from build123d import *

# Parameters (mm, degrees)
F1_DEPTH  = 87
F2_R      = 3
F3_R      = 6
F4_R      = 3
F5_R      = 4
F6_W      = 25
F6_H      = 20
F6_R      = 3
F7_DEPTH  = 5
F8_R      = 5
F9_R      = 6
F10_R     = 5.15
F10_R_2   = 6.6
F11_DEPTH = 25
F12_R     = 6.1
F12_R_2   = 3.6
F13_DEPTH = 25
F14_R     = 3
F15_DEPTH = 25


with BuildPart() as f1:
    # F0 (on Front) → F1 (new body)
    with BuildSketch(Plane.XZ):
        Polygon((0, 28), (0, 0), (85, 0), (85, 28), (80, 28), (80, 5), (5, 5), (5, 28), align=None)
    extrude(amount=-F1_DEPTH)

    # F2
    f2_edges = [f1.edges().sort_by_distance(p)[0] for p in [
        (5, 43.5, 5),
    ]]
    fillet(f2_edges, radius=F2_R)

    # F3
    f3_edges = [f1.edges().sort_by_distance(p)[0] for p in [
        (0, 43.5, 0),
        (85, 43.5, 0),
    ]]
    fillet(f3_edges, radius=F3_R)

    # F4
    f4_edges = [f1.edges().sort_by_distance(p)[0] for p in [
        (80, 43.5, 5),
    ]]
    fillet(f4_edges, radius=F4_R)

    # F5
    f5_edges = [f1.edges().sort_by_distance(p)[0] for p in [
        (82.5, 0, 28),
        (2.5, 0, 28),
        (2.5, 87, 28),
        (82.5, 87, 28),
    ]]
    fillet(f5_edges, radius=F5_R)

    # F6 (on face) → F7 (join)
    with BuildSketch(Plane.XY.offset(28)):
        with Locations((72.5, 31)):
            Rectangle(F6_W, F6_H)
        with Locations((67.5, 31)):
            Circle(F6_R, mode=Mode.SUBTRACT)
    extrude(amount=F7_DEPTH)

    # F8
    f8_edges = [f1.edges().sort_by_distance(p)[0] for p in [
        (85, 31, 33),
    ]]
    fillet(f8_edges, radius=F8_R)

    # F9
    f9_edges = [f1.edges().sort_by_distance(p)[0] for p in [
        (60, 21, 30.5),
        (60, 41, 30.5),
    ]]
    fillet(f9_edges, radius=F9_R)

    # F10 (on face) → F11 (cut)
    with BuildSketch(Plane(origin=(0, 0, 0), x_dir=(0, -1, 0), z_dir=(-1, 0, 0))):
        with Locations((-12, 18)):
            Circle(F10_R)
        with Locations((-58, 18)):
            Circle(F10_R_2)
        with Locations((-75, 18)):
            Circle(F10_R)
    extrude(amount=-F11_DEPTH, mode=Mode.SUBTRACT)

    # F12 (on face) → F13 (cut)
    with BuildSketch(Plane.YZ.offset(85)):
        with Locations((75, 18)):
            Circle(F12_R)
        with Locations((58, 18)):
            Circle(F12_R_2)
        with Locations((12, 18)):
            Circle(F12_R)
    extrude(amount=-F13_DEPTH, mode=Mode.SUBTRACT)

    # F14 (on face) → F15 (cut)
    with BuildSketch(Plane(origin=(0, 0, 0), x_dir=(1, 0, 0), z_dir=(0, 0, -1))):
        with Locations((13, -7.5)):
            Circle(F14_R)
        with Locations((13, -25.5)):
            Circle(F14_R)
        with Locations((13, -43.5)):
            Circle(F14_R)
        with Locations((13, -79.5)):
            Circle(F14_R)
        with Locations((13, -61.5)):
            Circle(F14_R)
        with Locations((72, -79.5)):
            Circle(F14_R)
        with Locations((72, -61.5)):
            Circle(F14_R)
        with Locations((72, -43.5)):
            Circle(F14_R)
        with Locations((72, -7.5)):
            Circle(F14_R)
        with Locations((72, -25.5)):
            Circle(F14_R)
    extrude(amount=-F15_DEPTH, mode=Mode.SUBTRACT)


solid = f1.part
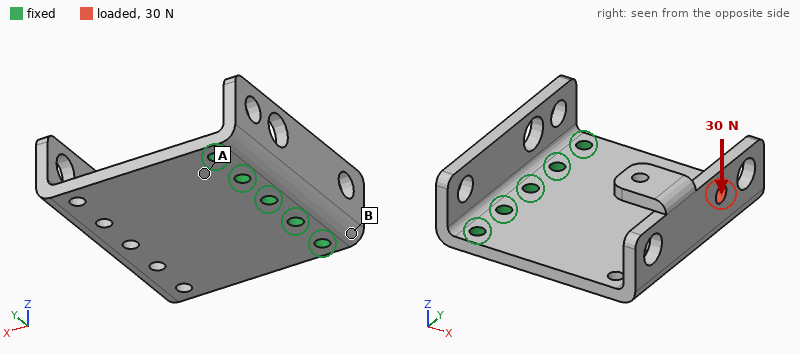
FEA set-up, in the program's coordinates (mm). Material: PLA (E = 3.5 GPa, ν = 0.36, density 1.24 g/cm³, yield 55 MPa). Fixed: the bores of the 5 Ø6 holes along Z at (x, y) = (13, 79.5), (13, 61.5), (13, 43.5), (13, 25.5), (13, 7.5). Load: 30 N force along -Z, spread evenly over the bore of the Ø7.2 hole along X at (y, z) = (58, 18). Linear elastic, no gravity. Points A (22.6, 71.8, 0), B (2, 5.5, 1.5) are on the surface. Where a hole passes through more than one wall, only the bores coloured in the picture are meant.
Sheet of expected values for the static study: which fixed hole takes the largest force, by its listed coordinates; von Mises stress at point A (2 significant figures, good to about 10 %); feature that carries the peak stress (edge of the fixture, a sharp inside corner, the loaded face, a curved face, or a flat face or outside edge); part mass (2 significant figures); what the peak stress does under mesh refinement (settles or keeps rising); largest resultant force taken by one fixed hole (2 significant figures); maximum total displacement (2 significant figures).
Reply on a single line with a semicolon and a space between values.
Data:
(13, 61.5); 4.9 MPa; edge of the fixture; 67 g; keeps rising; 14 N; 1.3 mm
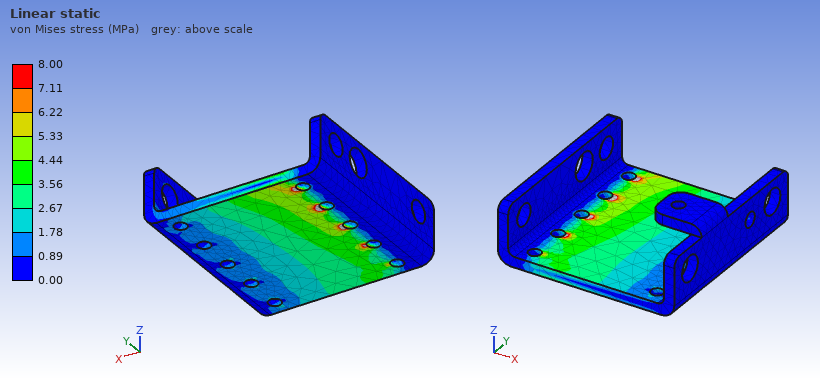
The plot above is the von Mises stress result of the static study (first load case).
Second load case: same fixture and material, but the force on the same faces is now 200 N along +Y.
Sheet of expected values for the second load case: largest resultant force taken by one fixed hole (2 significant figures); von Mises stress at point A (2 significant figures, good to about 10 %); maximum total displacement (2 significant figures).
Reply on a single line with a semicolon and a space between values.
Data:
170 N; 5.9 MPa; 1.4 mm
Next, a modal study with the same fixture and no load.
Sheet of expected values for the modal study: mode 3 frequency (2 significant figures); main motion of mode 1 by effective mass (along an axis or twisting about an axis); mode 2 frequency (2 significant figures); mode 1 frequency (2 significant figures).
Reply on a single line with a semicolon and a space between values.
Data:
710 Hz; along Z; 390 Hz; 190 Hz
